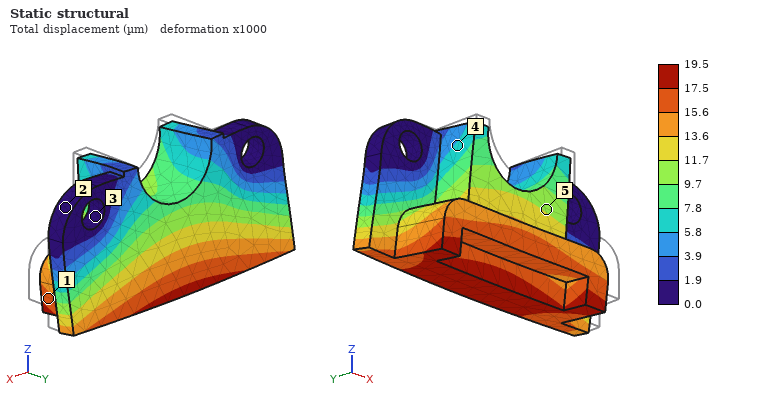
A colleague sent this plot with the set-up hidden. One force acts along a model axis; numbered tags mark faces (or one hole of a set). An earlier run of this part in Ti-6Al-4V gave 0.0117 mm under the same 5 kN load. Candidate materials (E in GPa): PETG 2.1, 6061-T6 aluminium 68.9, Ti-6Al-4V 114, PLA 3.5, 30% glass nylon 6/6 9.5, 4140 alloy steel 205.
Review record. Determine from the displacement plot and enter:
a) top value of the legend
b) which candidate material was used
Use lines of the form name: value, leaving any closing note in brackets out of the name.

top value of the legend: 19.5 µm
which candidate material was used: 6061-T6 aluminium
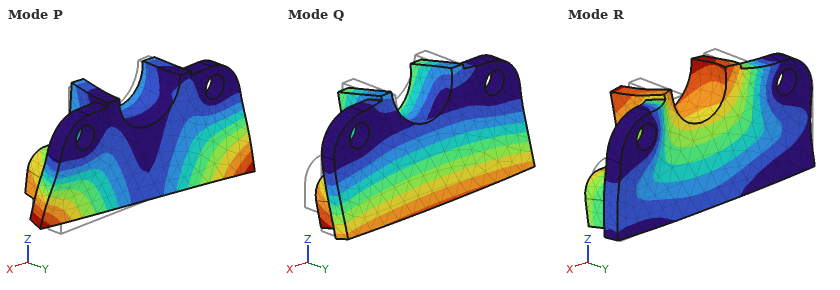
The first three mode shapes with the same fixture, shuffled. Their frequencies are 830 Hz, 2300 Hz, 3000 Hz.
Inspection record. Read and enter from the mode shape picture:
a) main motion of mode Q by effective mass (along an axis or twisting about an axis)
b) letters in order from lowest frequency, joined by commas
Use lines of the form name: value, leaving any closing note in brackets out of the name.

main motion of mode Q by effective mass: along Y
letters in order from lowest frequency, joined by commas: Q, P, R
